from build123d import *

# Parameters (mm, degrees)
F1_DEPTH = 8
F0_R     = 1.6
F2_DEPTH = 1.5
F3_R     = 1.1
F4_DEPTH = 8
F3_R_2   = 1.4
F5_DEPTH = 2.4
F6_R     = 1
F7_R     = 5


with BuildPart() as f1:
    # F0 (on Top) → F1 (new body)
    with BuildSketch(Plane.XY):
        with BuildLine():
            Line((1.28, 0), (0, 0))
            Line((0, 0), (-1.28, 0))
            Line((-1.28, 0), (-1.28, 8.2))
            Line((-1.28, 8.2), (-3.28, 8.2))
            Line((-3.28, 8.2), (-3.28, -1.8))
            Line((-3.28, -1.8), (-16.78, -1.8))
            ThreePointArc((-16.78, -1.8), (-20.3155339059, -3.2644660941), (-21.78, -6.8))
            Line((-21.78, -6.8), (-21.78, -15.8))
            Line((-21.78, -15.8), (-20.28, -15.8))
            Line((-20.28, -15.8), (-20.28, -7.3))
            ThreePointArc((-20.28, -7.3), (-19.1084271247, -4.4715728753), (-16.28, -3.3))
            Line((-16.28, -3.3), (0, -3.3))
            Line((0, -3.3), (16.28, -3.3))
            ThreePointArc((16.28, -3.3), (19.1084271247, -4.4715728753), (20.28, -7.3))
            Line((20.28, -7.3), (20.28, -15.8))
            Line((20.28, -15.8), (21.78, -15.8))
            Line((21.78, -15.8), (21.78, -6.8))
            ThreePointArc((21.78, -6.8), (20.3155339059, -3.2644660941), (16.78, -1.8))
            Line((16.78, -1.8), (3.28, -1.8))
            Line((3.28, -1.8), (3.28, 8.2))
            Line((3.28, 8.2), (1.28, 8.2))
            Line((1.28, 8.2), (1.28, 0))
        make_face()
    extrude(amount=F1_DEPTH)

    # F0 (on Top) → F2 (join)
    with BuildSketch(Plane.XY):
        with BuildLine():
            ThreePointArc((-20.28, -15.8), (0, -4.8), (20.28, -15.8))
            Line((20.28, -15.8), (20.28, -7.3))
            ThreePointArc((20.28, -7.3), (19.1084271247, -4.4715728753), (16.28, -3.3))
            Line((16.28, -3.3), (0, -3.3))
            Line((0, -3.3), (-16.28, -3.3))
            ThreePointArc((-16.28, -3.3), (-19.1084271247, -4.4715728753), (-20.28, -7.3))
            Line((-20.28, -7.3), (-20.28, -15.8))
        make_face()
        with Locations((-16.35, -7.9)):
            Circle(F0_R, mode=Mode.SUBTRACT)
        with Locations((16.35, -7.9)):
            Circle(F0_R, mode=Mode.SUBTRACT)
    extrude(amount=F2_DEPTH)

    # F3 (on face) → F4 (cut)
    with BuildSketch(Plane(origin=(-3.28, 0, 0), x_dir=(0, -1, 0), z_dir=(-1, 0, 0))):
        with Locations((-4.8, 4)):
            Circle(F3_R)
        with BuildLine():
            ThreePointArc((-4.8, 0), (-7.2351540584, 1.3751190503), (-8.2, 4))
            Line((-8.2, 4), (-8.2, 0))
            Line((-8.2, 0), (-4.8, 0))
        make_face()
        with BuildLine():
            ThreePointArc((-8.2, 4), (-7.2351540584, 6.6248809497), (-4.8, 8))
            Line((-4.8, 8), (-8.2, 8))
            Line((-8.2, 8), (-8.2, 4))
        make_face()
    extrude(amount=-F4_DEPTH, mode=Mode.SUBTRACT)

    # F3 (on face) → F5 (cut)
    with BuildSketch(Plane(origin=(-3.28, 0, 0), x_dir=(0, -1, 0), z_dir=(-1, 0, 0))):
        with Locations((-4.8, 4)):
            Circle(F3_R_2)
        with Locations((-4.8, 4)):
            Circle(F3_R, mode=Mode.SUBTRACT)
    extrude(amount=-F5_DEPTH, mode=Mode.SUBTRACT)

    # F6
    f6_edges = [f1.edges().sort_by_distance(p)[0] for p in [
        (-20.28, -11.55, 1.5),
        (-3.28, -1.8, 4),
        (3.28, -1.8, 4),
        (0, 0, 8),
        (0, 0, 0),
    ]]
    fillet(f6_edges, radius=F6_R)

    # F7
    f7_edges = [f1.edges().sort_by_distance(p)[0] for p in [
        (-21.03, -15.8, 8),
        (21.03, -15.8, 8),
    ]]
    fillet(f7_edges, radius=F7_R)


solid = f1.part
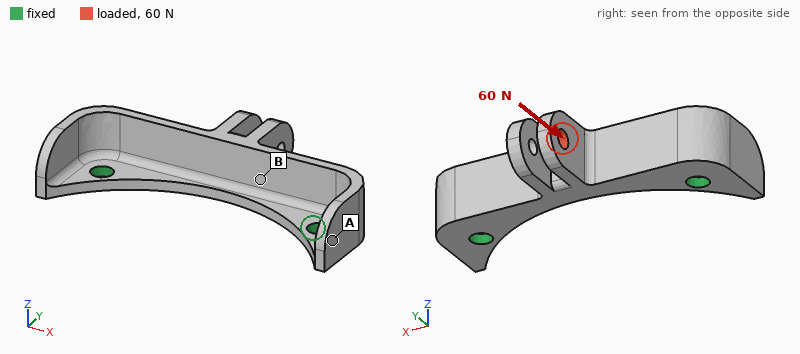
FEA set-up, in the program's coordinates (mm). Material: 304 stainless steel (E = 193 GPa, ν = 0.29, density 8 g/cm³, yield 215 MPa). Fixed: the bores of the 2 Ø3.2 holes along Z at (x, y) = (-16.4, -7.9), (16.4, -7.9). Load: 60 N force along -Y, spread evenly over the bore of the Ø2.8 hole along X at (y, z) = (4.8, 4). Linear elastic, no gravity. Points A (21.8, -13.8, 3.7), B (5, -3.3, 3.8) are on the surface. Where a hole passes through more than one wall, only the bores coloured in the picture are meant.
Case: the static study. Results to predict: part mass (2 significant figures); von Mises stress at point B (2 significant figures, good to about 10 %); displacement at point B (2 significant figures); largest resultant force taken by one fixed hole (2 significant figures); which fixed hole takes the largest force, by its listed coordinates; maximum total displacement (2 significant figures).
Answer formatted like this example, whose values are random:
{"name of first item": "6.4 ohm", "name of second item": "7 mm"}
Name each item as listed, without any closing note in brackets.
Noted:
{"part mass": "11 g", "von Mises stress at point B": "9.1 MPa", "displacement at point B": "4.2 µm", "largest resultant force taken by one fixed hole": "53 N", "which fixed hole takes the largest force, by its listed coordinates": "(-16.4, -7.9)", "maximum total displacement": "15 µm"}
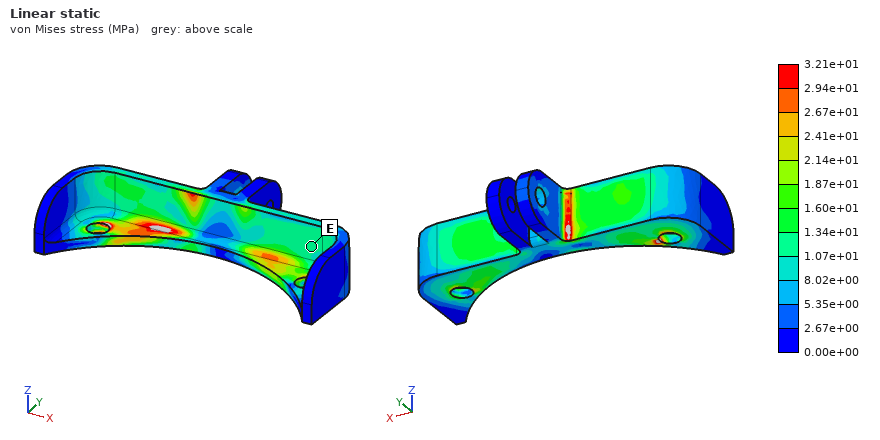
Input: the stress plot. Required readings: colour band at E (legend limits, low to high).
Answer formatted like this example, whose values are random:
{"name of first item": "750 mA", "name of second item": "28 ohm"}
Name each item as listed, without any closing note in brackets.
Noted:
{"colour band at E": "1.07e+01 to 1.34e+01 MPa"}
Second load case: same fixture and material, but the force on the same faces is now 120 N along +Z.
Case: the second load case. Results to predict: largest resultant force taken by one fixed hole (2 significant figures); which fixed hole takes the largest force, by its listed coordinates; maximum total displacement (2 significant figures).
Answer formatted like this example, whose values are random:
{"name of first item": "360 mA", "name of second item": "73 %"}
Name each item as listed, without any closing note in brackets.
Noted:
{"largest resultant force taken by one fixed hole": "89 N", "which fixed hole takes the largest force, by its listed coordinates": "(-16.4, -7.9)", "maximum total displacement": "87 µm"}
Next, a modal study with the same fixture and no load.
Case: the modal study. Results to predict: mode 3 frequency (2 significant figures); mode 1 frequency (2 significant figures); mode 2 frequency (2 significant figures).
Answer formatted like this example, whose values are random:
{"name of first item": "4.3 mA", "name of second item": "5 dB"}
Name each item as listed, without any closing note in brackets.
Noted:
{"mode 3 frequency": "14 kHz", "mode 1 frequency": "4500 Hz", "mode 2 frequency": "13 kHz"}
